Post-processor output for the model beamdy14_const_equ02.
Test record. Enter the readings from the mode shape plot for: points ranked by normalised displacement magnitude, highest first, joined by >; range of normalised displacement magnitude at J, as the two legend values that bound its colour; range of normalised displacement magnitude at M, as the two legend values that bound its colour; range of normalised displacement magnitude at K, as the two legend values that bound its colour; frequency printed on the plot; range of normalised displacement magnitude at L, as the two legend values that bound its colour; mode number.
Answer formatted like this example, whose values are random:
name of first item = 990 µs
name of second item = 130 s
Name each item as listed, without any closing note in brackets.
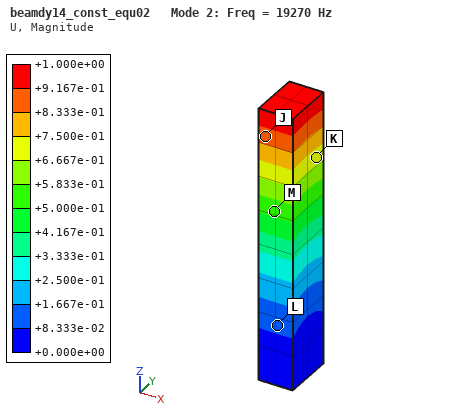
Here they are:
points ranked by normalised displacement magnitude, highest first, joined by > = J > K > M > L
range of normalised displacement magnitude at J, as the two legend values that bound its colour = +8.333e-01 to +9.167e-01
range of normalised displacement magnitude at M, as the two legend values that bound its colour = +5.000e-01 to +5.833e-01
range of normalised displacement magnitude at K, as the two legend values that bound its colour = +6.667e-01 to +7.500e-01
frequency printed on the plot = 19270 Hz
range of normalised displacement magnitude at L, as the two legend values that bound its colour = +8.333e-02 to +1.667e-01
mode number = 2
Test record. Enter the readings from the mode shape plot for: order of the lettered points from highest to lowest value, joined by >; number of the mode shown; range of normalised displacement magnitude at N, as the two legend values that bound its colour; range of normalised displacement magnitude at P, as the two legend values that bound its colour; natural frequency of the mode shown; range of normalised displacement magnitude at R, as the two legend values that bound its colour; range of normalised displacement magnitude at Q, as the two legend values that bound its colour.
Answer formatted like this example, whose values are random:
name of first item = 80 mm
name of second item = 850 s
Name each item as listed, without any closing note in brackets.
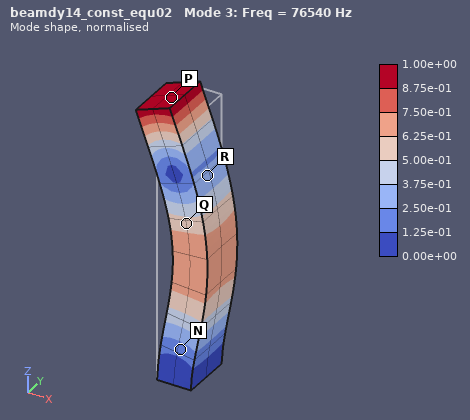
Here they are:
order of the lettered points from highest to lowest value, joined by > = P > Q > R > N
number of the mode shown = 3
range of normalised displacement magnitude at N, as the two legend values that bound its colour = 1.25e-01 to 2.50e-01
range of normalised displacement magnitude at P, as the two legend values that bound its colour = 8.75e-01 to 1.00e+00
natural frequency of the mode shown = 76540 Hz
range of normalised displacement magnitude at R, as the two legend values that bound its colour = 2.50e-01 to 3.75e-01
range of normalised displacement magnitude at Q, as the two legend values that bound its colour = 5.00e-01 to 6.25e-01
